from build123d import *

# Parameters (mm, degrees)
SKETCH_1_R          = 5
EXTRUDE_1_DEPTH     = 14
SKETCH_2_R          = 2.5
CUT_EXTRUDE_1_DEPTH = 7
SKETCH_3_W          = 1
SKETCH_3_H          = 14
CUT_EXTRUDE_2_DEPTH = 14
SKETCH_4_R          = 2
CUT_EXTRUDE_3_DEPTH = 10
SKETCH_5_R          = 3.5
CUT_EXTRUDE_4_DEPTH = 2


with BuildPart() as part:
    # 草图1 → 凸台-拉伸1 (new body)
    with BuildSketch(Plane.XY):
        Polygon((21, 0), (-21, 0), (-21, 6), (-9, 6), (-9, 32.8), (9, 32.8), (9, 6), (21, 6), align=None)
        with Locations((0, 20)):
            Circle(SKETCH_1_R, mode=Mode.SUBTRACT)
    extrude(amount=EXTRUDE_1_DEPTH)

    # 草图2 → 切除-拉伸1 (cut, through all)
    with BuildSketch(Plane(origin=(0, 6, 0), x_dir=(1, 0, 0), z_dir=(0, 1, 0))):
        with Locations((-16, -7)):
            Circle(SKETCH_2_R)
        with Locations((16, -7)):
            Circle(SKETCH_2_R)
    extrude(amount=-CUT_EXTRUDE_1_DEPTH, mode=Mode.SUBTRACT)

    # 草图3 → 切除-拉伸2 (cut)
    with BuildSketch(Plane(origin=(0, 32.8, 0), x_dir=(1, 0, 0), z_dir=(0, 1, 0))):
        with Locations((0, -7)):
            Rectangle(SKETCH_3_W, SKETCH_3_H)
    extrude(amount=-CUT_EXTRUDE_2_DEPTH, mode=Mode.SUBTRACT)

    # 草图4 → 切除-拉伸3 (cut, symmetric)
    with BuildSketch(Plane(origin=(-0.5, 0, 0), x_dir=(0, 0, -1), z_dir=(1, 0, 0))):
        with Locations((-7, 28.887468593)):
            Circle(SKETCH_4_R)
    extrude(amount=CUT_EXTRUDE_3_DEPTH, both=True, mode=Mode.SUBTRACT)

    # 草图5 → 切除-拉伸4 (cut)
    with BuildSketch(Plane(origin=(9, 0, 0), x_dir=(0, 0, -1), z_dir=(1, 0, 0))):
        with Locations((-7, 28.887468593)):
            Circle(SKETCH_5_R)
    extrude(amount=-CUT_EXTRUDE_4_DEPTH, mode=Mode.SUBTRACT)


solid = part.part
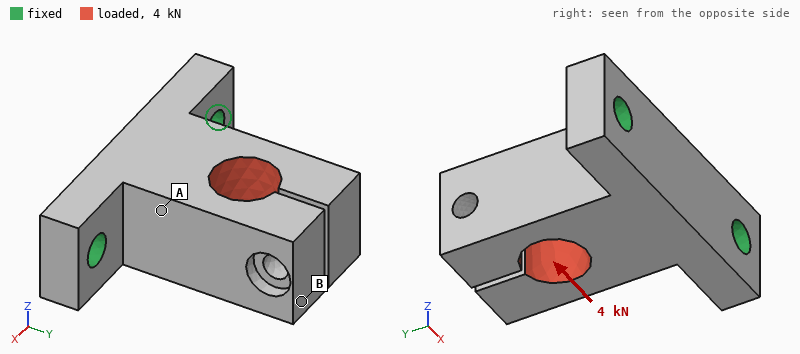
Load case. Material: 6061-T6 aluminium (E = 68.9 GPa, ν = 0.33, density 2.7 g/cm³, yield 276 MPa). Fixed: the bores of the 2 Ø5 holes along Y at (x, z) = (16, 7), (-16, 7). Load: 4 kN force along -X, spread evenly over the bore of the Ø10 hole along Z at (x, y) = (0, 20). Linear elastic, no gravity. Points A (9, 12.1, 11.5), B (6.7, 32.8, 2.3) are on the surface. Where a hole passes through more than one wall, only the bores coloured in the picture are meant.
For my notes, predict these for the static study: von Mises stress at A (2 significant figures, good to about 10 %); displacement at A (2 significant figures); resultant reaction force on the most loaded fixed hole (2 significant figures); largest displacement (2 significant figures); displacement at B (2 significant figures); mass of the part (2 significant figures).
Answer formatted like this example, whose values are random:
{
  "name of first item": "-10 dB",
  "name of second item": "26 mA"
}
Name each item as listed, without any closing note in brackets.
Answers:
{
  "von Mises stress at A": "75 MPa",
  "displacement at A": "0.031 mm",
  "resultant reaction force on the most loaded fixed hole": "3.4 kN",
  "largest displacement": "0.17 mm",
  "displacement at B": "0.17 mm",
  "mass of the part": "23 g"
}
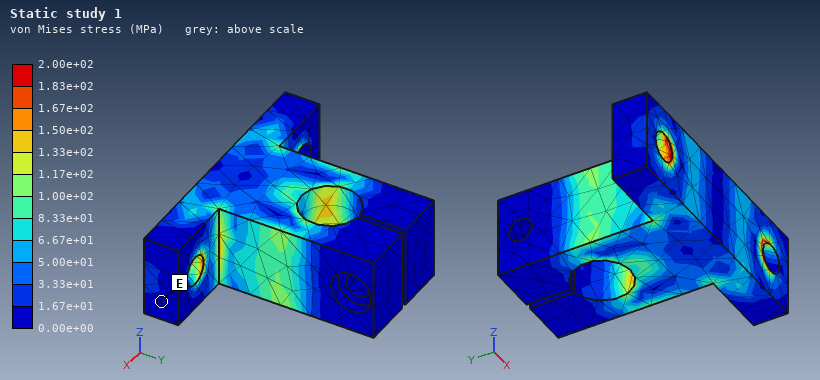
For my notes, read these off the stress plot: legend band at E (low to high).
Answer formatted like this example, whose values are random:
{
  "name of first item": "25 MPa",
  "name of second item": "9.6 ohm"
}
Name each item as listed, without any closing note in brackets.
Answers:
{
  "legend band at E": "0.00e+00 to 1.67e+01 MPa"
}
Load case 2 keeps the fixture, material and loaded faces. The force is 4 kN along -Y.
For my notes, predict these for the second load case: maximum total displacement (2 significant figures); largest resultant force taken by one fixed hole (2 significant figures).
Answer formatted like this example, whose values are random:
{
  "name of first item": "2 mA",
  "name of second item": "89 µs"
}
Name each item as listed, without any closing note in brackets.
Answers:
{
  "maximum total displacement": "86 µm",
  "largest resultant force taken by one fixed hole": "2.1 kN"
}
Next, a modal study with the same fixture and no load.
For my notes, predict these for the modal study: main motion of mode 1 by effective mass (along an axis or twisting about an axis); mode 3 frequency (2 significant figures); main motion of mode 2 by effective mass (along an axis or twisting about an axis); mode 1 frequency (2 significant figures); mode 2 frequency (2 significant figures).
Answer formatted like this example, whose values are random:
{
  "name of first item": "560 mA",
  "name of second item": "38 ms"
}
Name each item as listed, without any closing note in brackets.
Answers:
{
  "main motion of mode 1 by effective mass": "along Z",
  "mode 3 frequency": "7700 Hz",
  "main motion of mode 2 by effective mass": "along X",
  "mode 1 frequency": "5100 Hz",
  "mode 2 frequency": "6900 Hz"
}
